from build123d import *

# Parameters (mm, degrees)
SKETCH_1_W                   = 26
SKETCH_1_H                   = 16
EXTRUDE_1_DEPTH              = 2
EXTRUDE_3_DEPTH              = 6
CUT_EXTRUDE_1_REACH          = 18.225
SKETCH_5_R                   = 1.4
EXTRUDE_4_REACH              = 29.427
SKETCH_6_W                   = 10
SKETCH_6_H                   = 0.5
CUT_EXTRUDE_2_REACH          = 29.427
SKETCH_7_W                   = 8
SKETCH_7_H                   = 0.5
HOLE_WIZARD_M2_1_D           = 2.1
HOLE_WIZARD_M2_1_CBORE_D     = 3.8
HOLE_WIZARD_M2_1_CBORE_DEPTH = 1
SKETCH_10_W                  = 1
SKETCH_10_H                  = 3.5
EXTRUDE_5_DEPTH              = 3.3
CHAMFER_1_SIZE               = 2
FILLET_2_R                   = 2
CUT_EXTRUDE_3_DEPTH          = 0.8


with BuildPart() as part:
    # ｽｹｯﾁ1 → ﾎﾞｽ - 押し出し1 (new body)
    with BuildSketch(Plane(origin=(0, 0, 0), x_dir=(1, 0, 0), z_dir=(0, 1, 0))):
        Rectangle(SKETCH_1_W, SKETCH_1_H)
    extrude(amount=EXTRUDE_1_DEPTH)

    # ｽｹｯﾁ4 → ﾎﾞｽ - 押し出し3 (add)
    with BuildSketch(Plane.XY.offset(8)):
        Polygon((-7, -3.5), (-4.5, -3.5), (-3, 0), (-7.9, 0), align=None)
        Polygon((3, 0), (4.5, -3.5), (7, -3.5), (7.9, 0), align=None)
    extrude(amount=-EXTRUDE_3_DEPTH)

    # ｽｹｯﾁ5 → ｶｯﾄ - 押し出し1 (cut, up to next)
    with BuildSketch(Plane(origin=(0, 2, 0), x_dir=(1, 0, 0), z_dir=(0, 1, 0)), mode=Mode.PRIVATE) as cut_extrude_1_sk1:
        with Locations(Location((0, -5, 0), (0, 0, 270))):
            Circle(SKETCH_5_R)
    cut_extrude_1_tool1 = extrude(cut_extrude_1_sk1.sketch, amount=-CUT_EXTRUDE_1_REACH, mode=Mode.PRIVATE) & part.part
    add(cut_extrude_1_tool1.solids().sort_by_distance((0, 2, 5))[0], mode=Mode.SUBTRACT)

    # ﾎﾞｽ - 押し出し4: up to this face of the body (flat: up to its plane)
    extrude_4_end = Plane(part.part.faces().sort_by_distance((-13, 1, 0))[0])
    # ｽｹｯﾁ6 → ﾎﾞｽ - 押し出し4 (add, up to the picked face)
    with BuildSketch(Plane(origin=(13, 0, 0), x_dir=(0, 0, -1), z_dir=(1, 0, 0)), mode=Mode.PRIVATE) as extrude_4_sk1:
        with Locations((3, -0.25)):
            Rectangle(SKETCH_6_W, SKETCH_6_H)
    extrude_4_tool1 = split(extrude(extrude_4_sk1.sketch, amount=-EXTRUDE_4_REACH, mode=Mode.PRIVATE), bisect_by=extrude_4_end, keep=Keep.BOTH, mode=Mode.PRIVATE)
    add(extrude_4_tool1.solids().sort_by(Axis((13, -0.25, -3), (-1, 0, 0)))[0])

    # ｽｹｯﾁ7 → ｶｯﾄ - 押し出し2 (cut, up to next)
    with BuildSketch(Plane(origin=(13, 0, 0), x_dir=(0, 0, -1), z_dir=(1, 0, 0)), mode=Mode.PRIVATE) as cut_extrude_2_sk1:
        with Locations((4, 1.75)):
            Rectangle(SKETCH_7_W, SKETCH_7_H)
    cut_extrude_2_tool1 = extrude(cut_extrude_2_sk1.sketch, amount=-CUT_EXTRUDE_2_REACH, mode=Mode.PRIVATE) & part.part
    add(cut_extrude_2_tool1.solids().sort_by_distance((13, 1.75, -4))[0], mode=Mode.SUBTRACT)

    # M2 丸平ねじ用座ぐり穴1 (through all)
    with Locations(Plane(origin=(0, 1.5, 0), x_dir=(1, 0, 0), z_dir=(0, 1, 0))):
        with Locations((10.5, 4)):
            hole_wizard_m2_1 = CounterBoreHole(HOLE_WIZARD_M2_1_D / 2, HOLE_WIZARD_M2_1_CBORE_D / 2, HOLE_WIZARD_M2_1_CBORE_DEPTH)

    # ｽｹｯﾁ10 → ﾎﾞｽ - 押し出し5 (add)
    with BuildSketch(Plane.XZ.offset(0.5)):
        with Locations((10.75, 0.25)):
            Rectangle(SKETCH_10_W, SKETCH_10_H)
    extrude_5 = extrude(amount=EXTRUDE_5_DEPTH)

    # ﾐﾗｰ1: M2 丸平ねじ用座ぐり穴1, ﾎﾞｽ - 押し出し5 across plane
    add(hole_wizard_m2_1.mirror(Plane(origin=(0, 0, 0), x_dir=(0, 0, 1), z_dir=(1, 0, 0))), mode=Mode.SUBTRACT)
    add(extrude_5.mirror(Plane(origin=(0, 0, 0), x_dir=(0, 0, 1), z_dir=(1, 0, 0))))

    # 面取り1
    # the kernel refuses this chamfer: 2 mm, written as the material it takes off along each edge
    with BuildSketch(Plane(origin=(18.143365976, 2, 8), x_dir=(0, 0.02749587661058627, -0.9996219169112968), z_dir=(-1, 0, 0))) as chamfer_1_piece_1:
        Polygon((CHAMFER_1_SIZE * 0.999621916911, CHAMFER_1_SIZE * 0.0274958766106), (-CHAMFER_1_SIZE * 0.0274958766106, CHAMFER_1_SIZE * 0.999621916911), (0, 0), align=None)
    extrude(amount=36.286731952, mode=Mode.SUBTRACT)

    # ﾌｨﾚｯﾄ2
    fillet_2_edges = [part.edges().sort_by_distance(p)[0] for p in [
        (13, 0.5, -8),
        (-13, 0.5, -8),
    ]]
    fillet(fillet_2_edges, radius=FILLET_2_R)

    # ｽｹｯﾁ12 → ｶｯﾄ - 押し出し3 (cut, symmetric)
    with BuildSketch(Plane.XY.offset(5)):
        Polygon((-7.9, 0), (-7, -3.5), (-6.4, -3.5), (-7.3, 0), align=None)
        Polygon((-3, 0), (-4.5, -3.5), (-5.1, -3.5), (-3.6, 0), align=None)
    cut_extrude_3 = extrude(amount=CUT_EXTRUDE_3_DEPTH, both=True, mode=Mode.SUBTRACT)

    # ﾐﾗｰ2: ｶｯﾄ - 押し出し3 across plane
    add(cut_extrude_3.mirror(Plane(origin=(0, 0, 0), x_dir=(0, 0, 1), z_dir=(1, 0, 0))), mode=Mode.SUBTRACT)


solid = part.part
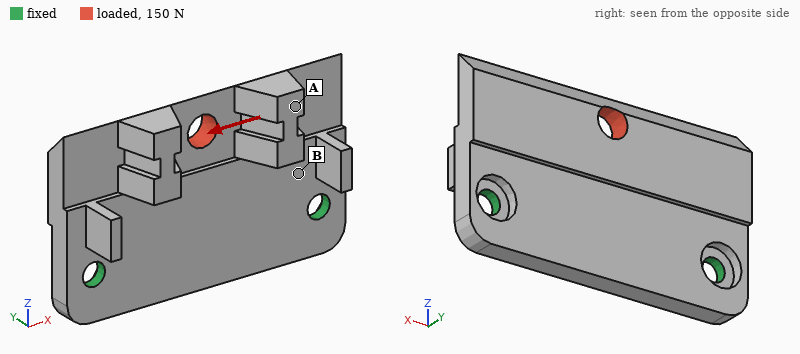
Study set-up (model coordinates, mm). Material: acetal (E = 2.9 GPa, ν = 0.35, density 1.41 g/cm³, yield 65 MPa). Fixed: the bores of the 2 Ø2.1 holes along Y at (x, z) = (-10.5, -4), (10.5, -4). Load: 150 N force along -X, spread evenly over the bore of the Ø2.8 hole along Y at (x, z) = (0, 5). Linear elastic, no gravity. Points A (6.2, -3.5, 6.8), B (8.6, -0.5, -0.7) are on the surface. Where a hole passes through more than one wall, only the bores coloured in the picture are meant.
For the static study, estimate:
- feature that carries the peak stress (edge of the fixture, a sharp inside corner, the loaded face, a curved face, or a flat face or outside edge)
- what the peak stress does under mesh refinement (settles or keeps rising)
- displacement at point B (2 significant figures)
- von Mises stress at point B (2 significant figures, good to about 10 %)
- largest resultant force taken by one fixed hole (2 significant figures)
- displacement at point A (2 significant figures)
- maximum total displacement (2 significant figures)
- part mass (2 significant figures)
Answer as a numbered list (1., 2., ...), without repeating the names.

1. edge of the fixture
2. keeps rising
3. 20 µm
4. 10 MPa
5. 97 N
6. 51 µm
7. 61 µm
8. 1.3 g
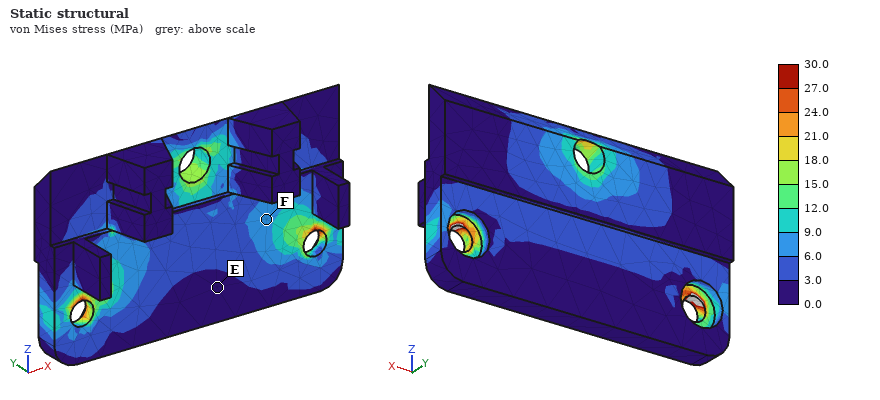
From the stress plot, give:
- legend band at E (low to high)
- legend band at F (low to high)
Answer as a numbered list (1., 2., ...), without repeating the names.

1. 0.0 to 3.0 MPa
2. 6.0 to 9.0 MPa
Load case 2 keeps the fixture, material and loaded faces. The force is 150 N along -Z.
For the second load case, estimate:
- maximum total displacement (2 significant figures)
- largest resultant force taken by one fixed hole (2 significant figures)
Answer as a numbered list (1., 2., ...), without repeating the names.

1. 0.33 mm
2. 80 N
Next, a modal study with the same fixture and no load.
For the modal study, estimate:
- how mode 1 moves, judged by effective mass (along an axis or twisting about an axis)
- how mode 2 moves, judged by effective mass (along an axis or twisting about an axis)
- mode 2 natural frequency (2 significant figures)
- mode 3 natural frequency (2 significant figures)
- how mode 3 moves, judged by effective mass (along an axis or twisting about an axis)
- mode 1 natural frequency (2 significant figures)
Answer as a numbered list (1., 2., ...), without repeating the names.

1. along Y
2. twisting about Z
3. 3900 Hz
4. 5100 Hz
5. along Y
6. 1700 Hz
